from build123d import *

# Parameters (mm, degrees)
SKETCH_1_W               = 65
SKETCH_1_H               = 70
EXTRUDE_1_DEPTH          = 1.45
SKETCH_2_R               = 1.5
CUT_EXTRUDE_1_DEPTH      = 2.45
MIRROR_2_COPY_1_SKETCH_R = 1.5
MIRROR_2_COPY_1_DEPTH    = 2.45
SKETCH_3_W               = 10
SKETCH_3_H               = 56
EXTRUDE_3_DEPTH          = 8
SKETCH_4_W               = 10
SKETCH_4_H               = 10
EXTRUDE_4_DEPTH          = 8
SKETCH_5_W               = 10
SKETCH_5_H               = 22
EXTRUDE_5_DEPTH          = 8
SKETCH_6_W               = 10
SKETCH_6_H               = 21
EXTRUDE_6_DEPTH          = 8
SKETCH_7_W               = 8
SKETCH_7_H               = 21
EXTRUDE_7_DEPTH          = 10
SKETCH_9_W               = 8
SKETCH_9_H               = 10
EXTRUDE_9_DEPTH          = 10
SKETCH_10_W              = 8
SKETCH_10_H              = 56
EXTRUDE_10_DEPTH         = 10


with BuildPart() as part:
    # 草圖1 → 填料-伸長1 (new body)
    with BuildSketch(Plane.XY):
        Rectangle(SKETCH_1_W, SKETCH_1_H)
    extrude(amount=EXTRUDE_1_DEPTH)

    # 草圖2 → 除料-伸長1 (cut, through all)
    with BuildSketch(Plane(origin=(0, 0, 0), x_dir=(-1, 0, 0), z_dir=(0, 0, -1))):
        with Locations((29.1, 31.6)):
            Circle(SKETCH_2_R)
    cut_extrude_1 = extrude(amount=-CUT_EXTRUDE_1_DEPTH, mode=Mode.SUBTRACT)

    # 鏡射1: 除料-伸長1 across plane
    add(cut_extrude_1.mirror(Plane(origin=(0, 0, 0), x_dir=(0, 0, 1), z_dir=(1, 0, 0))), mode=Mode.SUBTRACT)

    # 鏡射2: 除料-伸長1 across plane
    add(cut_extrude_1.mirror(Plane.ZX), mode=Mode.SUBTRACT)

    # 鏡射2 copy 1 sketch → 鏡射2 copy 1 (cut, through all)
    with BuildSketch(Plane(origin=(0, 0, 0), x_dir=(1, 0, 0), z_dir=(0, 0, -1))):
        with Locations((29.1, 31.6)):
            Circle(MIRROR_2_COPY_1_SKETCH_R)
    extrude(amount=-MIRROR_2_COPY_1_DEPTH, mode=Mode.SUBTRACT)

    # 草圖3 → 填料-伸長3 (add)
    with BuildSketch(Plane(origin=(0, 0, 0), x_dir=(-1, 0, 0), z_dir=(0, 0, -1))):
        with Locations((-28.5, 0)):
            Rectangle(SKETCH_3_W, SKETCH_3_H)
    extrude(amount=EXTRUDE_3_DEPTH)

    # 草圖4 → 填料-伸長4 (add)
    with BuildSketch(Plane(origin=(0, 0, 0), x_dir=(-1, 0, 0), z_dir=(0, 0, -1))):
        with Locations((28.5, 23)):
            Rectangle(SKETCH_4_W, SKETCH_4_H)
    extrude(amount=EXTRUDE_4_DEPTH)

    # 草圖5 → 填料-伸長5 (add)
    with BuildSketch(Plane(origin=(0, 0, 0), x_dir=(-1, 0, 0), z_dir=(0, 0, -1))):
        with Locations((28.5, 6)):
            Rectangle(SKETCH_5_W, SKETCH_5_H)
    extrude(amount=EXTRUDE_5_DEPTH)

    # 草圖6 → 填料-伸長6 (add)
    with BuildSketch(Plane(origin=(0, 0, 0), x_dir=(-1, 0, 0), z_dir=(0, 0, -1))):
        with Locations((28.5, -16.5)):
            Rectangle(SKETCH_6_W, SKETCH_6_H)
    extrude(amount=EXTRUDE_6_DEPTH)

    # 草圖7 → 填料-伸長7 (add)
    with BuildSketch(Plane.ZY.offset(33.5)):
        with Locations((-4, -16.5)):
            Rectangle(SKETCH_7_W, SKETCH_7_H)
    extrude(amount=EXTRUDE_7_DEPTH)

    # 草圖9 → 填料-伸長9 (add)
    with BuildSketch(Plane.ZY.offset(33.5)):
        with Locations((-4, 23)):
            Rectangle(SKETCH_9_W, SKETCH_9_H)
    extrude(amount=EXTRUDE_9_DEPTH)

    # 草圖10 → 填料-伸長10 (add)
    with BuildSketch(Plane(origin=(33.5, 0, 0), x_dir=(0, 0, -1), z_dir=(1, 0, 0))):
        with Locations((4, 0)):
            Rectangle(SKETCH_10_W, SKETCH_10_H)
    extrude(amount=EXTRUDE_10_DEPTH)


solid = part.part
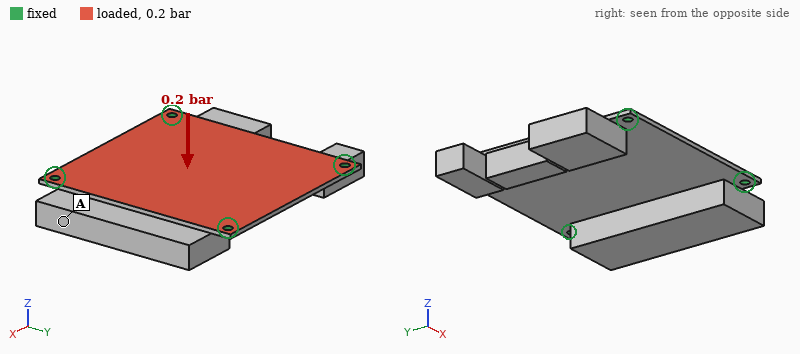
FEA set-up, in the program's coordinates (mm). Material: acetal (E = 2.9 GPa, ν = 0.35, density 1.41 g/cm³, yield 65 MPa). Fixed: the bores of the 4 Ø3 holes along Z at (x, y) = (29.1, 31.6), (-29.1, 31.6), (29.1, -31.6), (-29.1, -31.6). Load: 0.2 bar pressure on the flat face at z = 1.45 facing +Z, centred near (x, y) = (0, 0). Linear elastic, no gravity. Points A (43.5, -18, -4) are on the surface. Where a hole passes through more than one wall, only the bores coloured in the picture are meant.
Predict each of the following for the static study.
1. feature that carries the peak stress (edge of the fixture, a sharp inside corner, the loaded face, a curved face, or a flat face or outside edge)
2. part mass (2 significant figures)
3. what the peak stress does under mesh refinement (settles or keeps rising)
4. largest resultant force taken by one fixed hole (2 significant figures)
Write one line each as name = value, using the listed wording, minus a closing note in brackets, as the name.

feature that carries the peak stress = edge of the fixture
part mass = 31 g
what the peak stress does under mesh refinement = keeps rising
largest resultant force taken by one fixed hole = 31 N
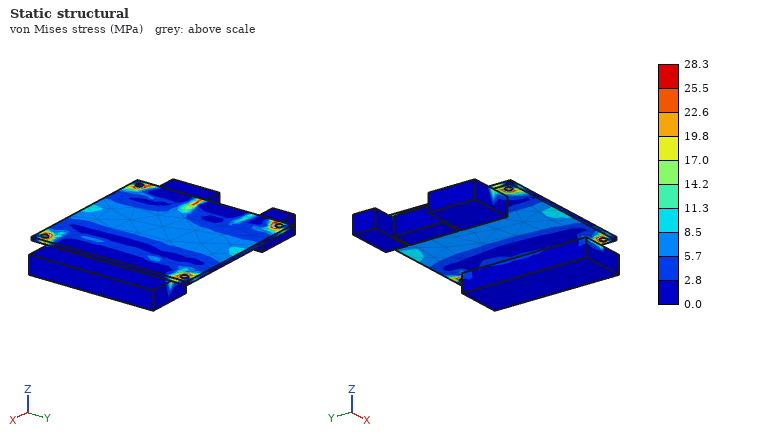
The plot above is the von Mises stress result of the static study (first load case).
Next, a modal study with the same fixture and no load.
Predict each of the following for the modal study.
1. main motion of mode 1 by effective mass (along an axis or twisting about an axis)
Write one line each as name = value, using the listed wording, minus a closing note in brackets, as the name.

main motion of mode 1 by effective mass = along Z
